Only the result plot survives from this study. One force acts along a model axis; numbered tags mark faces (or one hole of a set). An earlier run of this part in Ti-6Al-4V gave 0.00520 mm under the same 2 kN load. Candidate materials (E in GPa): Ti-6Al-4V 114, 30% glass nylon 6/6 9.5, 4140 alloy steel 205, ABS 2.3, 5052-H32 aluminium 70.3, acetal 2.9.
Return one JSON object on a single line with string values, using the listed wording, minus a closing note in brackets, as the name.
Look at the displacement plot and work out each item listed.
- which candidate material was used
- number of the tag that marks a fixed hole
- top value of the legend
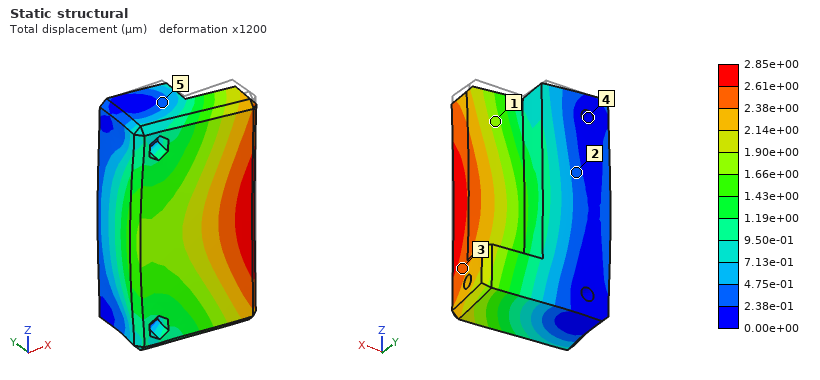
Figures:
{"which candidate material was used": "4140 alloy steel", "number of the tag that marks a fixed hole": "4", "top value of the legend": "2.85e+00 µm"}
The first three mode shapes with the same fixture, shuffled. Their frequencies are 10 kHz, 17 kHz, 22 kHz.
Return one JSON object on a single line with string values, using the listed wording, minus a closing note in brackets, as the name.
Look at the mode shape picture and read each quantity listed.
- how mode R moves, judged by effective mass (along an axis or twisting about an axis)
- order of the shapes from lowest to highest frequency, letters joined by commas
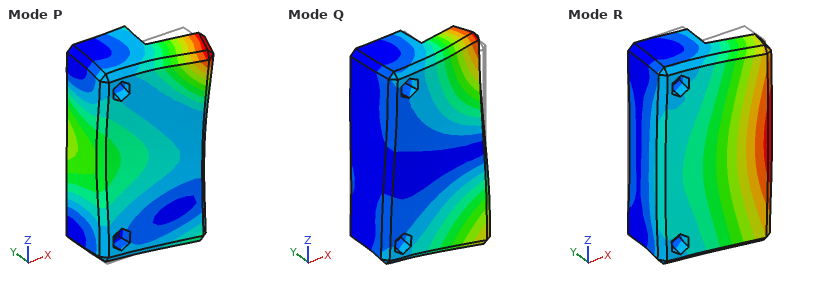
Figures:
{"how mode R moves, judged by effective mass": "along Y", "order of the shapes from lowest to highest frequency, letters joined by commas": "R, Q, P"}
